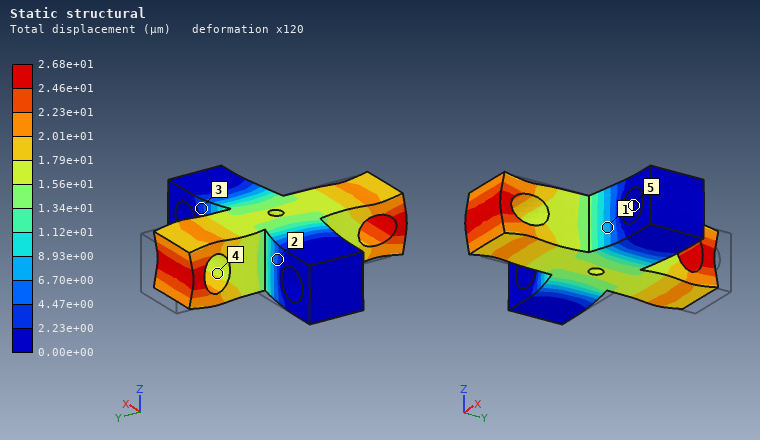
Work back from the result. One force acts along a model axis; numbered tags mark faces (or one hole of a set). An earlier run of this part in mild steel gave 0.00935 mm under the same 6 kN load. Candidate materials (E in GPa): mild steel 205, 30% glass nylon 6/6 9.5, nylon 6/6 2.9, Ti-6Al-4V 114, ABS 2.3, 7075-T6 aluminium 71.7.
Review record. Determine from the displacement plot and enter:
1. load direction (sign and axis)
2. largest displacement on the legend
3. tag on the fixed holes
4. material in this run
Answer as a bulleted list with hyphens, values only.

- -Y
- 2.68e+01 µm
- 5
- 7075-T6 aluminium
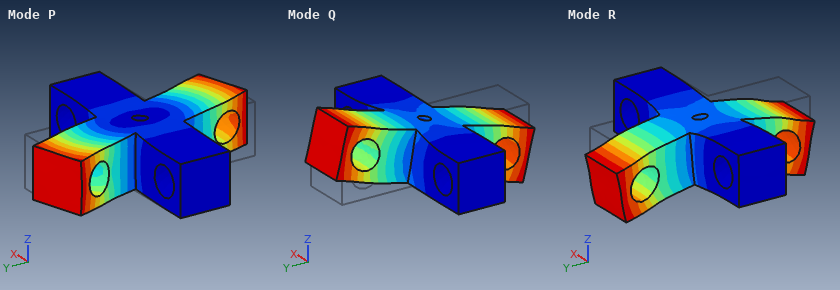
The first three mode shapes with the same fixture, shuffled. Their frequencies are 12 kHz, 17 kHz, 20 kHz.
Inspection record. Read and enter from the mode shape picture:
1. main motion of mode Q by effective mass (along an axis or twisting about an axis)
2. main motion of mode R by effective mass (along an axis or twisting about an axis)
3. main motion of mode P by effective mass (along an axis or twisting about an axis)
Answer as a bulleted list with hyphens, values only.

- twisting about X
- along Z
- twisting about Z
